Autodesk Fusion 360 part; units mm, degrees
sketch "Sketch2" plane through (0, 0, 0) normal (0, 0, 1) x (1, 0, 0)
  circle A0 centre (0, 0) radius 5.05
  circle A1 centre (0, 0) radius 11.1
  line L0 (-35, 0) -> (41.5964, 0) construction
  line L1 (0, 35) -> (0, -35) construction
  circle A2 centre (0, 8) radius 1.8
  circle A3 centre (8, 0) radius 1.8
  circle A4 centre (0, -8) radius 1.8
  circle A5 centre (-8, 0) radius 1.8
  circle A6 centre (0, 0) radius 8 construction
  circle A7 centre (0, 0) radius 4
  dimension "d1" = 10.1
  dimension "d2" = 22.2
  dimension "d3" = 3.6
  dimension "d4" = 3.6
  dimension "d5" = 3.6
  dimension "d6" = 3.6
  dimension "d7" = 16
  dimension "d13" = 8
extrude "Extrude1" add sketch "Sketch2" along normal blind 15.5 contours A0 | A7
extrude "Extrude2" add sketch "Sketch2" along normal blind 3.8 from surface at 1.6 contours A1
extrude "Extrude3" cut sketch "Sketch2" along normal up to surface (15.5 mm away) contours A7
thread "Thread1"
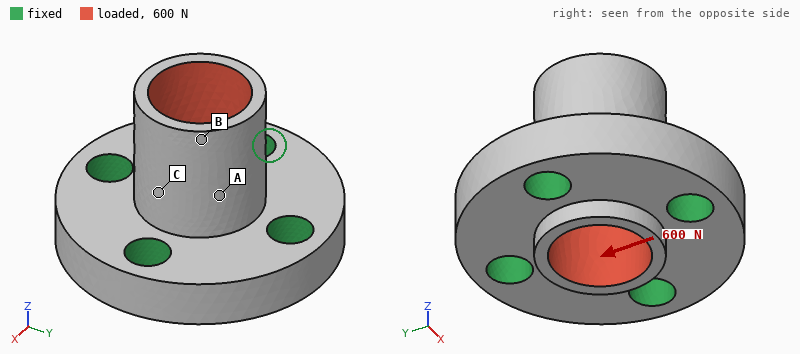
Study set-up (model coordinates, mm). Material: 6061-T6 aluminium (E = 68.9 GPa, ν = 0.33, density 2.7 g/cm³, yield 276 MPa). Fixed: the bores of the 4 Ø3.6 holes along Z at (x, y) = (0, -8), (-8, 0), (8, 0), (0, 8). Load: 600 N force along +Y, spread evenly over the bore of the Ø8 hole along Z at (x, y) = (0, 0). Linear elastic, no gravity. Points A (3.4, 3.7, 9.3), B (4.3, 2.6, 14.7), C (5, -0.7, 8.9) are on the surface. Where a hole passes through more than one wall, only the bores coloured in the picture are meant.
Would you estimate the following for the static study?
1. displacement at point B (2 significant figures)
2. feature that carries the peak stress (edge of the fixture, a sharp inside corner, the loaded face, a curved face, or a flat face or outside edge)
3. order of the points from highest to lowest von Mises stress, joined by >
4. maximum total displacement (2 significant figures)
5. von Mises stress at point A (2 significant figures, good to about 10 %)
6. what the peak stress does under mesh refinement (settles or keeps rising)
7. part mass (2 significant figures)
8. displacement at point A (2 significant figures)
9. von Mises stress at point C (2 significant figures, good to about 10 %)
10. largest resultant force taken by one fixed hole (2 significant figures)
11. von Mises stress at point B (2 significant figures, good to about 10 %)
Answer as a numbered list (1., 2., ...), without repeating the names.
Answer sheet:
1. 9.5 µm
2. a sharp inside corner
3. C > A > B
4. 11 µm
5. 19 MPa
6. keeps rising
7. 4.0 g
8. 5.4 µm
9. 25 MPa
10. 250 N
11. 4.5 MPa
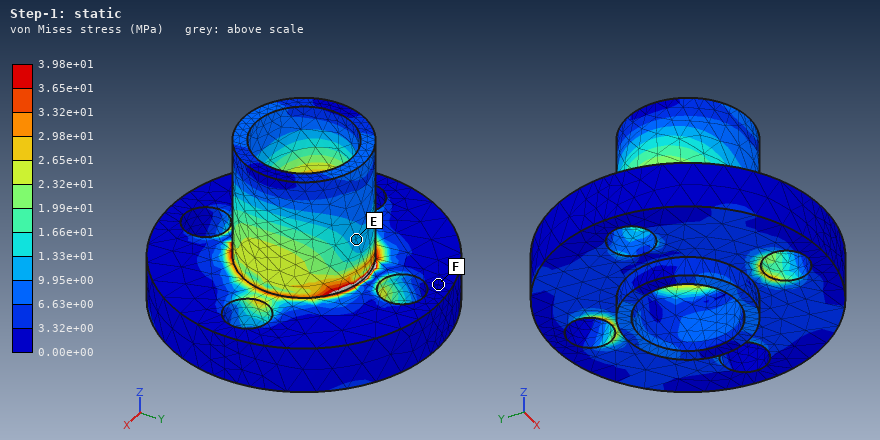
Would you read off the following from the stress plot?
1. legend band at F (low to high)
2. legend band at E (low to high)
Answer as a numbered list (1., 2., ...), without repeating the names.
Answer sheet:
1. 0.00e+00 to 3.32e+00 MPa
2. 9.95e+00 to 1.33e+01 MPa
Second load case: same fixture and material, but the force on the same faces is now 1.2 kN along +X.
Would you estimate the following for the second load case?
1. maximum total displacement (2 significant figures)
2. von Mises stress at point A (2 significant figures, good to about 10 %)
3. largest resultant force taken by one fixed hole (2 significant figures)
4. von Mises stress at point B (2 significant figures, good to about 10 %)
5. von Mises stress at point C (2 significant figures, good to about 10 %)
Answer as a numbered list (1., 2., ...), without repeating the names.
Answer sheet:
1. 21 µm
2. 39 MPa
3. 500 N
4. 12 MPa
5. 23 MPa
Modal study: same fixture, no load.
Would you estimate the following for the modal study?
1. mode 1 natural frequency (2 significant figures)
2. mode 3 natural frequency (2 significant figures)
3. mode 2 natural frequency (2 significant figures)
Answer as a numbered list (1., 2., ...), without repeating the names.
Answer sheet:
1. 39 kHz
2. 41 kHz
3. 39 kHz
